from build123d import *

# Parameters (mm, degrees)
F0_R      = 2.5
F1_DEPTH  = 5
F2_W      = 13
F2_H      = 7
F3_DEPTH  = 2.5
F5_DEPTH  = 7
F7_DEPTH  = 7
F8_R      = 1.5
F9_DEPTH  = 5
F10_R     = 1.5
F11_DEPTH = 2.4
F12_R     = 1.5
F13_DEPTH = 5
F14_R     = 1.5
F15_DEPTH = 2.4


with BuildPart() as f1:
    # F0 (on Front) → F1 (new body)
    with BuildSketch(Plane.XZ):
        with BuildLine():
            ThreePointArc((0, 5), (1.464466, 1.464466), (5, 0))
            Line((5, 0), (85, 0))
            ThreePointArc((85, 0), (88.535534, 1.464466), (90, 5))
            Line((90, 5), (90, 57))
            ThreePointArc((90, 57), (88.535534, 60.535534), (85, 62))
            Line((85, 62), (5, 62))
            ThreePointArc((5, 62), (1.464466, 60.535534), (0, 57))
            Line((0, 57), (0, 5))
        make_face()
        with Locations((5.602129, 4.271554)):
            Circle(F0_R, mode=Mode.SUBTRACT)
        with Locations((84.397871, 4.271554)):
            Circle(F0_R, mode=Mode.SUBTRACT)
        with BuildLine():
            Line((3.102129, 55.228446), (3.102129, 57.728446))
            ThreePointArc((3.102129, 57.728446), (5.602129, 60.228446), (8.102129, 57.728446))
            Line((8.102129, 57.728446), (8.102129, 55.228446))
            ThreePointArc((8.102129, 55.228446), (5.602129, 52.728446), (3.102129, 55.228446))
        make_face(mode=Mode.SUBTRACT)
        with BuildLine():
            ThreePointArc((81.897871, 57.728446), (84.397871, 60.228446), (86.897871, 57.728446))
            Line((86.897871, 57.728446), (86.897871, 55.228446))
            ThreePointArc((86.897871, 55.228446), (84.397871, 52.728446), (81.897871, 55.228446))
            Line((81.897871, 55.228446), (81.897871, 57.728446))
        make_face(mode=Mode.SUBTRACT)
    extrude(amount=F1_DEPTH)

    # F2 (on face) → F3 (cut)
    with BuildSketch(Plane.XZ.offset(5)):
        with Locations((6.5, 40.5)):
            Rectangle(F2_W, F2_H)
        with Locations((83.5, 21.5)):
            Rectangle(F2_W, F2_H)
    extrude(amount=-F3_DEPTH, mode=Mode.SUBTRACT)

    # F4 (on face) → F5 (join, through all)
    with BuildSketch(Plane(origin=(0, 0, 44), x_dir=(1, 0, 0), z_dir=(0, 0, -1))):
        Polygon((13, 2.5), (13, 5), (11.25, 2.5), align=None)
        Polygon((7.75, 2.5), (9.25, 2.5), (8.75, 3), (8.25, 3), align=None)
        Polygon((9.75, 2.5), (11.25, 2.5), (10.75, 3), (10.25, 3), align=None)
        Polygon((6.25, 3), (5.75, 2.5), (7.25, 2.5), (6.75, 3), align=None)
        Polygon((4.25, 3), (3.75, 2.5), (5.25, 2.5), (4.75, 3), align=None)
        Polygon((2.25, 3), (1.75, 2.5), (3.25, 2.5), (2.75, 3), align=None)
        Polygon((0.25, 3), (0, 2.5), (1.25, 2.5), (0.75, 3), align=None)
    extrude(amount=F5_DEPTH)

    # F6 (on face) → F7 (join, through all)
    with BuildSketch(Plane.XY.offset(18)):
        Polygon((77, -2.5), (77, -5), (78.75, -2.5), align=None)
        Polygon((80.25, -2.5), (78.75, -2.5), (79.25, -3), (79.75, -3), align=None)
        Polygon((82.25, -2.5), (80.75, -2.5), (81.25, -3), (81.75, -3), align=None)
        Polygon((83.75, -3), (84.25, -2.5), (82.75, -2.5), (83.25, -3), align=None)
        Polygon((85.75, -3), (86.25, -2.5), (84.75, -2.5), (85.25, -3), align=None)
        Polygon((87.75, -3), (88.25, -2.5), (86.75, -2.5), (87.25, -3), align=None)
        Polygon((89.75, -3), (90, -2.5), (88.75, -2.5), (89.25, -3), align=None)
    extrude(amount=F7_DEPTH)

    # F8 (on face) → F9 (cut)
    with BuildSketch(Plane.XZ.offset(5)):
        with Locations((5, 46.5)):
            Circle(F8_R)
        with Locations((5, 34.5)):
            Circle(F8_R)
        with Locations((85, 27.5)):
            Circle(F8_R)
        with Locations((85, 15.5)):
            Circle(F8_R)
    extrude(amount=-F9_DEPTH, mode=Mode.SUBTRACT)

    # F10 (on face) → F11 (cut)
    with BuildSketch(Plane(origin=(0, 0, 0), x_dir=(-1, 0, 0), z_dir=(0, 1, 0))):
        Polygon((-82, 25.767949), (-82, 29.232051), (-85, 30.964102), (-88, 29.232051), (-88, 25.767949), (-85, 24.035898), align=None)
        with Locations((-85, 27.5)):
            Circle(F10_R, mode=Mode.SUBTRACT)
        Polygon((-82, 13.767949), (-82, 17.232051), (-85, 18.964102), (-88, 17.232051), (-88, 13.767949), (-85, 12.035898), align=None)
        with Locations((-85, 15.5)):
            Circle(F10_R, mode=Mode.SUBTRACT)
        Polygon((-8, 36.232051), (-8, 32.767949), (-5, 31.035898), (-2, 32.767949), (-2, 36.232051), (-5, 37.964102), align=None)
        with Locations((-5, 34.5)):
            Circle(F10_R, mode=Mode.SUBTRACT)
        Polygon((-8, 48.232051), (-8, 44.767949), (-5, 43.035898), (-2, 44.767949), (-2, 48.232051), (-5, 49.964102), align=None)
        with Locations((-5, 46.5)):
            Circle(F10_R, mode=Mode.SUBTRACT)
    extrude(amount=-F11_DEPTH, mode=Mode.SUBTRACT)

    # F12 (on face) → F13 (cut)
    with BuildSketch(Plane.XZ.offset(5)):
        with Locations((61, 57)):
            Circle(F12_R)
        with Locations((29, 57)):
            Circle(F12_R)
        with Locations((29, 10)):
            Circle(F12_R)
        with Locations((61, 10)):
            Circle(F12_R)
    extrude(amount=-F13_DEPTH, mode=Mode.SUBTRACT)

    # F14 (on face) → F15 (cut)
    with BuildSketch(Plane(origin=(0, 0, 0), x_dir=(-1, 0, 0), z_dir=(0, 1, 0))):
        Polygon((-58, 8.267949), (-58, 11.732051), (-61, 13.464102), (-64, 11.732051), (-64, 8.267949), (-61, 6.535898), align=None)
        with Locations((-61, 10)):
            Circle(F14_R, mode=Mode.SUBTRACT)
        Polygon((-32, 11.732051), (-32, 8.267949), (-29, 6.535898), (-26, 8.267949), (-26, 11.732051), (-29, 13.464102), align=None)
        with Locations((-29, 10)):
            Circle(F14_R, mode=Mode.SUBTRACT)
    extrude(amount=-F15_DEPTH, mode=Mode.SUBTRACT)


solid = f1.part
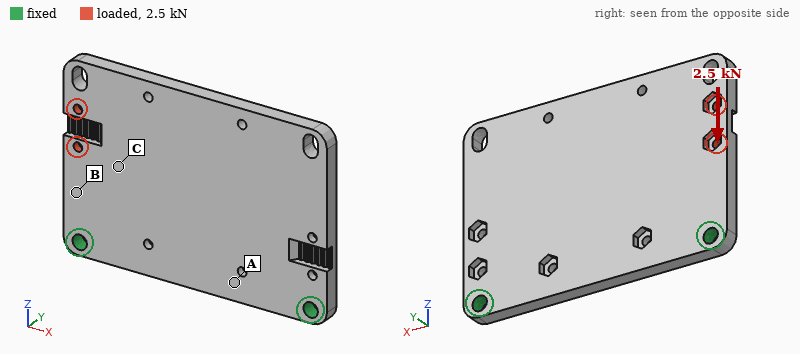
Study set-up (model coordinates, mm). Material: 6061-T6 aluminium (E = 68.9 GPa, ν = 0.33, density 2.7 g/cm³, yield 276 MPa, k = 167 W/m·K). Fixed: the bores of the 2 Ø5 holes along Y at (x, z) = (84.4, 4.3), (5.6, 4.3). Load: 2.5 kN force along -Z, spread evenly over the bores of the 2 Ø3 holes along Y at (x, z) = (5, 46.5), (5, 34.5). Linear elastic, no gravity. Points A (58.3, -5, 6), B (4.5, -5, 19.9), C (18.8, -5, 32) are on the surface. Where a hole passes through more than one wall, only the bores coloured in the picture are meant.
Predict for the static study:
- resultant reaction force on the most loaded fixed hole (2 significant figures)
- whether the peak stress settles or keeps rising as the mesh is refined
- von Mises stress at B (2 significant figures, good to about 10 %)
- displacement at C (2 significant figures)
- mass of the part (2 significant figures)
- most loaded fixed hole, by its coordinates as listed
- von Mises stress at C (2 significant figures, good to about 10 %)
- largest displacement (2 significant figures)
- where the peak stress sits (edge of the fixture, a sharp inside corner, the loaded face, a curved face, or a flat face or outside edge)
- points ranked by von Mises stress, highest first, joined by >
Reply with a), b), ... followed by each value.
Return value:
a) 2.5 kN
b) keeps rising
c) 51 MPa
d) 0.050 mm
e) 71 g
f) (5.6, 4.3)
g) 22 MPa
h) 0.18 mm
i) a sharp inside corner
j) B > C > A
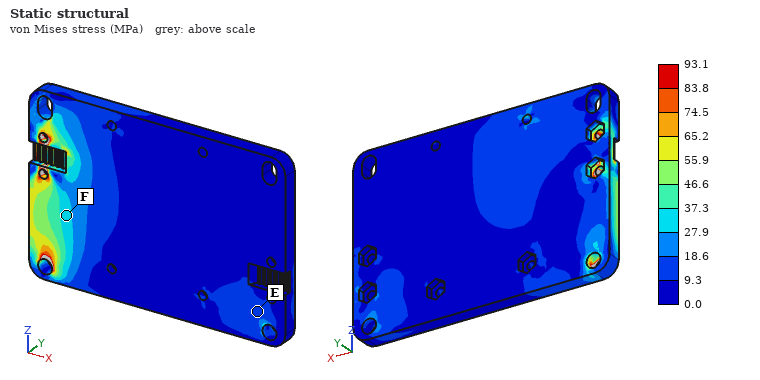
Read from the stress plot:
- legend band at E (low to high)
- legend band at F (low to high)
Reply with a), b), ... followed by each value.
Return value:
a) 9.3 to 18.6 MPa
b) 27.9 to 37.3 MPa
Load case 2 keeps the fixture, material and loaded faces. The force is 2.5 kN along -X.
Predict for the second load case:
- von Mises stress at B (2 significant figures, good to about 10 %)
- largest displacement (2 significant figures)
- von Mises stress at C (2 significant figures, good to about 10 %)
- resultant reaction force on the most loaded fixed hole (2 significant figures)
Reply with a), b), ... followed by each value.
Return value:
a) 20 MPa
b) 51 µm
c) 28 MPa
d) 1.7 kN
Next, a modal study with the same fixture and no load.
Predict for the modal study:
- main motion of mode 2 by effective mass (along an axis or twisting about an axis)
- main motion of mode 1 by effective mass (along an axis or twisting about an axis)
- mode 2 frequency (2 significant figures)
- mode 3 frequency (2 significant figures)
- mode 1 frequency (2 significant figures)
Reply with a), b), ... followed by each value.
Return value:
a) twisting about Z
b) along Y
c) 2200 Hz
d) 3800 Hz
e) 850 Hz
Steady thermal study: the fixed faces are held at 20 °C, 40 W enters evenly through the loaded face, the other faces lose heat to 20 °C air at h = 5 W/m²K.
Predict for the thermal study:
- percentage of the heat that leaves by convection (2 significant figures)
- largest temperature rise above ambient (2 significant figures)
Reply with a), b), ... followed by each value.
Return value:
a) 3.8 %
b) 70 K
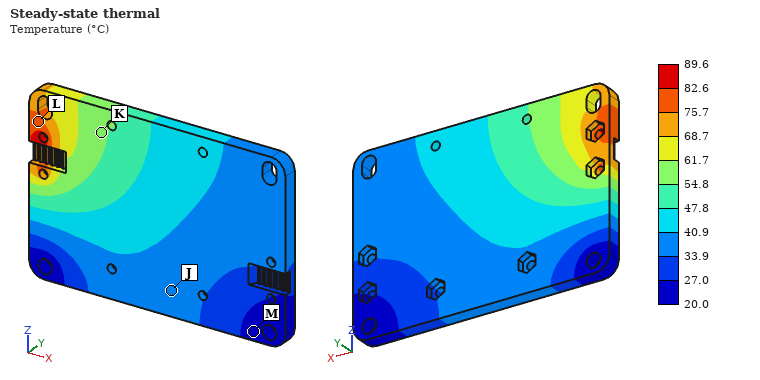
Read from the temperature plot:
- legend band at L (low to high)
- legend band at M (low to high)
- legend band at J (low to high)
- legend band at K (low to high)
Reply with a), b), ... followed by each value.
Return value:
a) 75.7 to 82.6 °C
b) 20.0 to 27.0 °C
c) 33.9 to 40.9 °C
d) 54.8 to 61.7 °C
